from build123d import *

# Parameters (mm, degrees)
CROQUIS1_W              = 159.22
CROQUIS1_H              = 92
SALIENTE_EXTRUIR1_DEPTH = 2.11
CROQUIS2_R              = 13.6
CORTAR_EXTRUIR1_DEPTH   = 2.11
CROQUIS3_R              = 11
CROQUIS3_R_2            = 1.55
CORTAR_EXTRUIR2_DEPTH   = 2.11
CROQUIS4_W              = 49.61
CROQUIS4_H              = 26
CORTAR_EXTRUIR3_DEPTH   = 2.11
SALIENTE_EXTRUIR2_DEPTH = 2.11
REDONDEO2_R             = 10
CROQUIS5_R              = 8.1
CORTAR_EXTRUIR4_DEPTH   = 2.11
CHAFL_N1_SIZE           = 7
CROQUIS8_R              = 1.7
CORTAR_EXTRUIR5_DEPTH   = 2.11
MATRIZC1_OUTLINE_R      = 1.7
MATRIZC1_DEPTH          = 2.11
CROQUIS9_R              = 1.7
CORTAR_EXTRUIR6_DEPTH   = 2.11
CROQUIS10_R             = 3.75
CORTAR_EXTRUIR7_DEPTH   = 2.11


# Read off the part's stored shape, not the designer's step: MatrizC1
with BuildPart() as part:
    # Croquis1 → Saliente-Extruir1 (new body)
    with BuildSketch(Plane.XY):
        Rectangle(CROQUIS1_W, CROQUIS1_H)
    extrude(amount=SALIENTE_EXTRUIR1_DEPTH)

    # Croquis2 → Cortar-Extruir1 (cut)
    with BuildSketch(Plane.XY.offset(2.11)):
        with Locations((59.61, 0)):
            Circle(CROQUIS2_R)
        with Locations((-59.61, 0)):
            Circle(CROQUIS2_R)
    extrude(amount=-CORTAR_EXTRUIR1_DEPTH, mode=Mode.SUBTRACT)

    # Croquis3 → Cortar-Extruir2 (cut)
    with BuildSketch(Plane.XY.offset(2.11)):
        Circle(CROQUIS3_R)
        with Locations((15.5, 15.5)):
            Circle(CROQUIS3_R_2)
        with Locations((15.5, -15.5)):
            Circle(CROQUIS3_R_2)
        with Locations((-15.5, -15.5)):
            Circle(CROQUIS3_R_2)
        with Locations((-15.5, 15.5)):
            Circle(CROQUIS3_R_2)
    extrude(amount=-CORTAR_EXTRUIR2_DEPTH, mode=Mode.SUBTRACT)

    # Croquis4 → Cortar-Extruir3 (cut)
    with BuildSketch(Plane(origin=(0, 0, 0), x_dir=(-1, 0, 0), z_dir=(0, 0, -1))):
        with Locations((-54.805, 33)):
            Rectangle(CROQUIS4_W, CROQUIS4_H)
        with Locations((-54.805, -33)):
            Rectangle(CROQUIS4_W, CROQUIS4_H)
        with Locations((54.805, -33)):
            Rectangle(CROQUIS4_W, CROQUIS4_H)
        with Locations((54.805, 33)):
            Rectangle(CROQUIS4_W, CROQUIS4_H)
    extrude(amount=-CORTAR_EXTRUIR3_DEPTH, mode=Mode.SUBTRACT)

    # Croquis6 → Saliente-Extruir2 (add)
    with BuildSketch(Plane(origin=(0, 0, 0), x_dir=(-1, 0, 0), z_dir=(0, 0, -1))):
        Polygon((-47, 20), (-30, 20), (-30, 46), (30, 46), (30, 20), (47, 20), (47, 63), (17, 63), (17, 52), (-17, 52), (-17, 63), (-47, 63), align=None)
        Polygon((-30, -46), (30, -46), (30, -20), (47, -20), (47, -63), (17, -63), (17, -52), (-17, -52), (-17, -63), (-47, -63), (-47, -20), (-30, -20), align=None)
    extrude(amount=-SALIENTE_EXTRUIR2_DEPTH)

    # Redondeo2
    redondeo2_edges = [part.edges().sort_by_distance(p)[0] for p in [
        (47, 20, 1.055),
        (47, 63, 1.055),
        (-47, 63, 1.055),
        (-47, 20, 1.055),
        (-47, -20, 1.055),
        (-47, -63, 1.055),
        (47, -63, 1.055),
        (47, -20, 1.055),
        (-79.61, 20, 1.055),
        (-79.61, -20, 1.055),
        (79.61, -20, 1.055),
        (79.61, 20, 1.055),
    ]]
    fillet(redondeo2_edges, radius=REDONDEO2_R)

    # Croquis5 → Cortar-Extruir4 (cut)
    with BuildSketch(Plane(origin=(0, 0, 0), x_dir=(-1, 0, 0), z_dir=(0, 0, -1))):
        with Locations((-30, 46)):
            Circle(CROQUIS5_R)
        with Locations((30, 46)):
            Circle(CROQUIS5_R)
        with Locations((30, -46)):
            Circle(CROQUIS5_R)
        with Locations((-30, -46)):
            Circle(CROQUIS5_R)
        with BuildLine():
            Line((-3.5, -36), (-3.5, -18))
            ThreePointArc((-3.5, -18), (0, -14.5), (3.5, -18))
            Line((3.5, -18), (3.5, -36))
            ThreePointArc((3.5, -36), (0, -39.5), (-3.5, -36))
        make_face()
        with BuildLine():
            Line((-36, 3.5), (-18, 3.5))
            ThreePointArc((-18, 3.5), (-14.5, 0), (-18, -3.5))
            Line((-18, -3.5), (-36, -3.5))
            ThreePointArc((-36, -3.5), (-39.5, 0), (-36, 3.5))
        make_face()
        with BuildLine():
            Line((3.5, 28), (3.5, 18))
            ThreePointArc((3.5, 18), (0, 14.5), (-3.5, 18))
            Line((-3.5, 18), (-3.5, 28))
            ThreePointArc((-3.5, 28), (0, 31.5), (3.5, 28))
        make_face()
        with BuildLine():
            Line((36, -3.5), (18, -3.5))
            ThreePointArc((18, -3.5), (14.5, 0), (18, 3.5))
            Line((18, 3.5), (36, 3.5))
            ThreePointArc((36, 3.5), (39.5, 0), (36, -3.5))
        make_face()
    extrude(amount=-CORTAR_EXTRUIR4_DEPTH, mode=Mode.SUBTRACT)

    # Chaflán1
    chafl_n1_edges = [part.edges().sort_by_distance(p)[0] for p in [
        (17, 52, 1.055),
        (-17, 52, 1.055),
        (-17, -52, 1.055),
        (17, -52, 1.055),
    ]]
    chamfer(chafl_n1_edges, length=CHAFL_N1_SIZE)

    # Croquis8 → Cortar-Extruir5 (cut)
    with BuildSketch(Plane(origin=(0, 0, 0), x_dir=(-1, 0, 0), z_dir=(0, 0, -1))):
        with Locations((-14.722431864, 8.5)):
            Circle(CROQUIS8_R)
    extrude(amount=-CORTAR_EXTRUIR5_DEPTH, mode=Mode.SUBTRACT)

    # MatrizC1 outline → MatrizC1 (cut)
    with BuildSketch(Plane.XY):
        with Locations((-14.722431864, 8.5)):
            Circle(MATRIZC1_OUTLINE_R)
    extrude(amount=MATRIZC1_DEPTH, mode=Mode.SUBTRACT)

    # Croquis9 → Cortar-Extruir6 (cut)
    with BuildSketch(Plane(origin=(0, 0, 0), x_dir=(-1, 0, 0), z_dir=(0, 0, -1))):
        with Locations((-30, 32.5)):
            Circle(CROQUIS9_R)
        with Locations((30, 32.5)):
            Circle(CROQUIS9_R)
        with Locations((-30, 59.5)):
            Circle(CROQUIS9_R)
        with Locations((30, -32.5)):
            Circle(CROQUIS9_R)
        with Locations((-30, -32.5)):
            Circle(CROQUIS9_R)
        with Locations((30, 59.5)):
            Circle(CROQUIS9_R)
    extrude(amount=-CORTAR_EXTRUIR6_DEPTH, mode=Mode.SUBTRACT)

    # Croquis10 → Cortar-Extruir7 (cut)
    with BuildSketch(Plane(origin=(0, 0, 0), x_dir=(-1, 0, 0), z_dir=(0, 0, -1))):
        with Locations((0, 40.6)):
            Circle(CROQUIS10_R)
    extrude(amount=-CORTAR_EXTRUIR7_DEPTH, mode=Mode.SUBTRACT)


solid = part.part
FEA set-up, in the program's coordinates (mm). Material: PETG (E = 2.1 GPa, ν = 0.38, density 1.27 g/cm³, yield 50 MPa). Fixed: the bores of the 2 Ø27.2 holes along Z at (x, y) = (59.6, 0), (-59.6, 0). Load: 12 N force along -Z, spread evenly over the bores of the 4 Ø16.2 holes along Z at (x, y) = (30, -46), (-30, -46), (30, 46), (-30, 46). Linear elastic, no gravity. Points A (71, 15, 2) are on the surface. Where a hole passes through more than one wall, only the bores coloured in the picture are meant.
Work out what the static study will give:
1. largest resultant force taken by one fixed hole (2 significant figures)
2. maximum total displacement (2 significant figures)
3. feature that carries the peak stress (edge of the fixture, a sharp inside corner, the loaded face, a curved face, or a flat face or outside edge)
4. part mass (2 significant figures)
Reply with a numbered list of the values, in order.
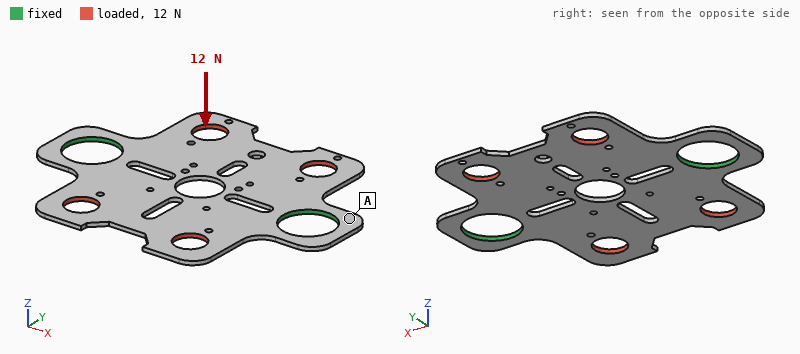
1. 6.0 N
2. 2.1 mm
3. a curved face
4. 28 g
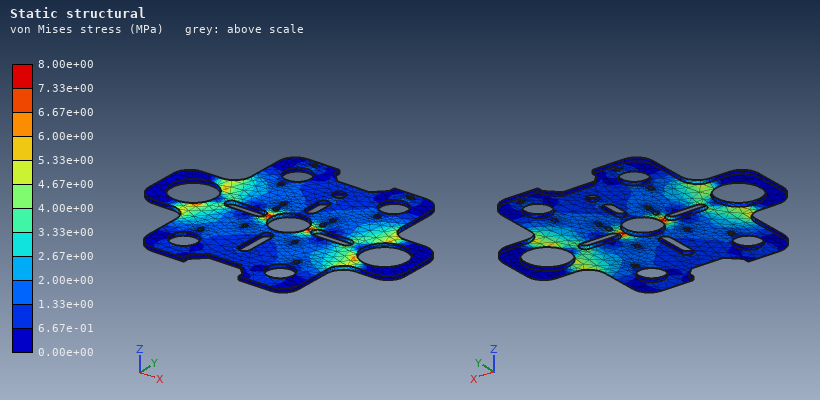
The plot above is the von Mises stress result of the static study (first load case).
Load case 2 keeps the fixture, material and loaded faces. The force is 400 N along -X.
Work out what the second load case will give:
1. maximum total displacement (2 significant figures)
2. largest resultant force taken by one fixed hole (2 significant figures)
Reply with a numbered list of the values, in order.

1. 0.12 mm
2. 200 N
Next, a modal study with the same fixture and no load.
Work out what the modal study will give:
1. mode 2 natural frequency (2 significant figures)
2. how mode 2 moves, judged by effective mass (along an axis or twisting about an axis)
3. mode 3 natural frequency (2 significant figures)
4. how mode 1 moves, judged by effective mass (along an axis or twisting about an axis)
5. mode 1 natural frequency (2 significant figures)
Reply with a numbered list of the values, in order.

1. 130 Hz
2. along Z
3. 250 Hz
4. twisting about X
5. 120 Hz
